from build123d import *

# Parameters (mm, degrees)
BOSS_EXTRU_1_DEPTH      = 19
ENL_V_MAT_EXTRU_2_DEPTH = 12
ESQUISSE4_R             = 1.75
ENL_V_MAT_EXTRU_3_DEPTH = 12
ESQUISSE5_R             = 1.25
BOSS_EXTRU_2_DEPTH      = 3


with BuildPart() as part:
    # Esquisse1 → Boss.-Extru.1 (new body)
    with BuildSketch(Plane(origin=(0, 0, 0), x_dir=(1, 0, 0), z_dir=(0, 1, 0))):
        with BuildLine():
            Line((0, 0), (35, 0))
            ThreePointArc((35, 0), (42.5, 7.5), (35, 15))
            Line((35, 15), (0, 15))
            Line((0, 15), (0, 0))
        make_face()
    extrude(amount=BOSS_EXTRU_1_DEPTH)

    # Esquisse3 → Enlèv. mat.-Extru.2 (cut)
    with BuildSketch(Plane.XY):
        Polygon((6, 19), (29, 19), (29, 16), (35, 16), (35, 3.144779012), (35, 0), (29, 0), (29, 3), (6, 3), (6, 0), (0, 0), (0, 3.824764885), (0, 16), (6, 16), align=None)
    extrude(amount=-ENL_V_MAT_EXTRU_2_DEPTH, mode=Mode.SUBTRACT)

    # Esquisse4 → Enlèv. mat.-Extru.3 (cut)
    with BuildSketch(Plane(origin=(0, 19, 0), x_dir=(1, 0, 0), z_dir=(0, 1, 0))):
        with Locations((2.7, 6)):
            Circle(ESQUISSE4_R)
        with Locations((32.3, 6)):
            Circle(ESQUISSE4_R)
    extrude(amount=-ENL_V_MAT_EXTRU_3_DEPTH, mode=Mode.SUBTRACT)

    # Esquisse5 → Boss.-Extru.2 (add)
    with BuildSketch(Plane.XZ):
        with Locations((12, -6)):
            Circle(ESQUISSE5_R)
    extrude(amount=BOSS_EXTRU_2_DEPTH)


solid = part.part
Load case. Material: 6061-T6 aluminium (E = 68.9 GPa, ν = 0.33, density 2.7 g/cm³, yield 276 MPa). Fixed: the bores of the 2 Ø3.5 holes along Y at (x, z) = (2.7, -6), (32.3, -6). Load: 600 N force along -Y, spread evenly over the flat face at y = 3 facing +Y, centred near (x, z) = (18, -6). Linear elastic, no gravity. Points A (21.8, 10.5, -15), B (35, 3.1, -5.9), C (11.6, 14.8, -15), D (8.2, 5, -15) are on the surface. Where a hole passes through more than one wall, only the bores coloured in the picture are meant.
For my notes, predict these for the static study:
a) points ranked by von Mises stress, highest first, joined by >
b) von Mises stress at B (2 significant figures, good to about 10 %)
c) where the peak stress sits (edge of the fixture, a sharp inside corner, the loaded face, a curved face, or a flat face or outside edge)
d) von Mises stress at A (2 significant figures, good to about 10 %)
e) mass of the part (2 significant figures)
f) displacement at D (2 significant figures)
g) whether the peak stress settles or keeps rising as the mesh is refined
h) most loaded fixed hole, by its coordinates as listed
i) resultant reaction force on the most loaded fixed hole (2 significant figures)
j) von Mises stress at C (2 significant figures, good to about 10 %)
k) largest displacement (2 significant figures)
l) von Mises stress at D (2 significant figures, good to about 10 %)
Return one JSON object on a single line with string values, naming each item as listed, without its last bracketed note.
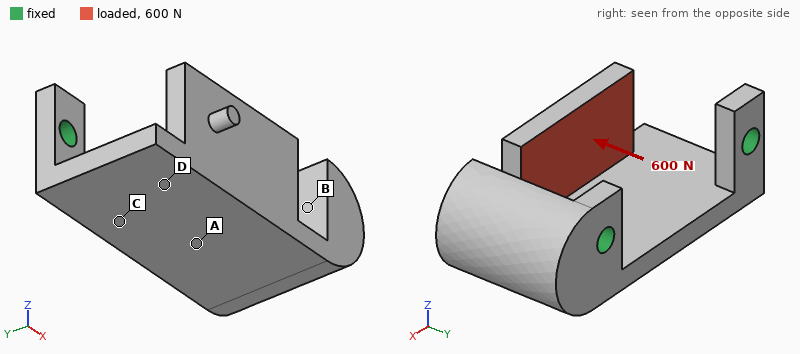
{"points ranked by von Mises stress, highest first, joined by >": "D > A > C > B", "von Mises stress at B": "15 MPa", "where the peak stress sits": "a sharp inside corner", "von Mises stress at A": "44 MPa", "mass of the part": "13 g", "displacement at D": "0.069 mm", "whether the peak stress settles or keeps rising as the mesh is refined": "keeps rising", "most loaded fixed hole, by its coordinates as listed": "(2.7, -6)", "resultant reaction force on the most loaded fixed hole": "320 N", "von Mises stress at C": "26 MPa", "largest displacement": "0.25 mm", "von Mises stress at D": "66 MPa"}
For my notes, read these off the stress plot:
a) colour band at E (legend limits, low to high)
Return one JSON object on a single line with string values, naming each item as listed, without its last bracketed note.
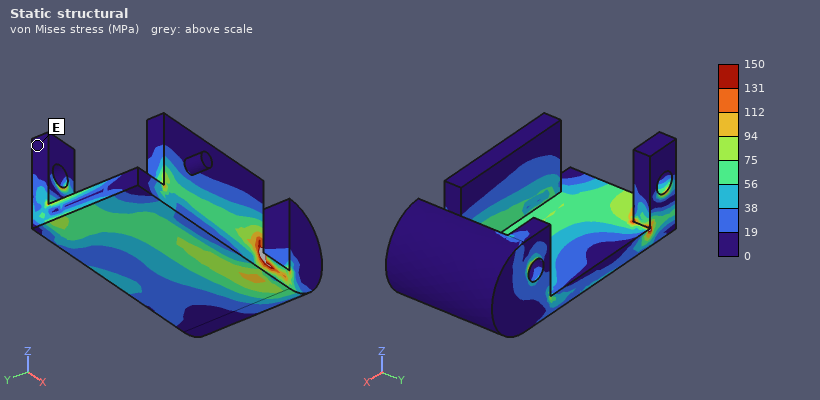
{"colour band at E": "0 to 19 MPa"}
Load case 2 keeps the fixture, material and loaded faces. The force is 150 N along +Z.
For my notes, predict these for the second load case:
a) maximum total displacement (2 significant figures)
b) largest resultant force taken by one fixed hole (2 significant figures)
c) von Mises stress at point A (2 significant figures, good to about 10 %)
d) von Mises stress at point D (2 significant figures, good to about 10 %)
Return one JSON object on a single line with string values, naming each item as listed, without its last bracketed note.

{"maximum total displacement": "92 µm", "largest resultant force taken by one fixed hole": "82 N", "von Mises stress at point A": "15 MPa", "von Mises stress at point D": "18 MPa"}
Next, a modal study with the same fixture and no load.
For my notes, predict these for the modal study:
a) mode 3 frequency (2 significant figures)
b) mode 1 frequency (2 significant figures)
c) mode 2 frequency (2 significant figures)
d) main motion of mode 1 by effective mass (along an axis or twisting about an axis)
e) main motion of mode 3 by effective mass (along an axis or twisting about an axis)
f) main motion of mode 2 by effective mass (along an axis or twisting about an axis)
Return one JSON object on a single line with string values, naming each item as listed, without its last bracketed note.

{"mode 3 frequency": "7700 Hz", "mode 1 frequency": "3300 Hz", "mode 2 frequency": "5800 Hz", "main motion of mode 1 by effective mass": "along Z", "main motion of mode 3 by effective mass": "along Y", "main motion of mode 2 by effective mass": "along X"}
